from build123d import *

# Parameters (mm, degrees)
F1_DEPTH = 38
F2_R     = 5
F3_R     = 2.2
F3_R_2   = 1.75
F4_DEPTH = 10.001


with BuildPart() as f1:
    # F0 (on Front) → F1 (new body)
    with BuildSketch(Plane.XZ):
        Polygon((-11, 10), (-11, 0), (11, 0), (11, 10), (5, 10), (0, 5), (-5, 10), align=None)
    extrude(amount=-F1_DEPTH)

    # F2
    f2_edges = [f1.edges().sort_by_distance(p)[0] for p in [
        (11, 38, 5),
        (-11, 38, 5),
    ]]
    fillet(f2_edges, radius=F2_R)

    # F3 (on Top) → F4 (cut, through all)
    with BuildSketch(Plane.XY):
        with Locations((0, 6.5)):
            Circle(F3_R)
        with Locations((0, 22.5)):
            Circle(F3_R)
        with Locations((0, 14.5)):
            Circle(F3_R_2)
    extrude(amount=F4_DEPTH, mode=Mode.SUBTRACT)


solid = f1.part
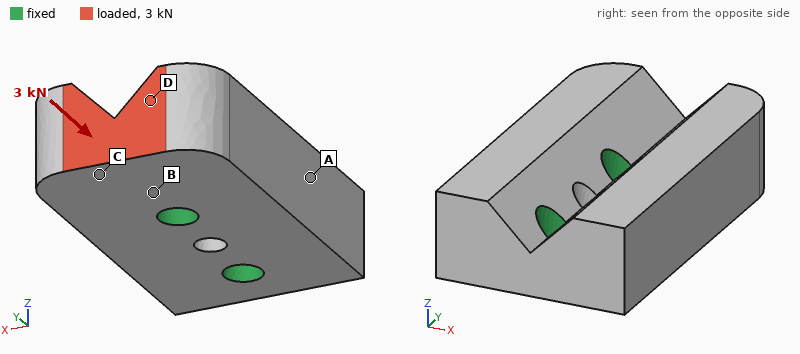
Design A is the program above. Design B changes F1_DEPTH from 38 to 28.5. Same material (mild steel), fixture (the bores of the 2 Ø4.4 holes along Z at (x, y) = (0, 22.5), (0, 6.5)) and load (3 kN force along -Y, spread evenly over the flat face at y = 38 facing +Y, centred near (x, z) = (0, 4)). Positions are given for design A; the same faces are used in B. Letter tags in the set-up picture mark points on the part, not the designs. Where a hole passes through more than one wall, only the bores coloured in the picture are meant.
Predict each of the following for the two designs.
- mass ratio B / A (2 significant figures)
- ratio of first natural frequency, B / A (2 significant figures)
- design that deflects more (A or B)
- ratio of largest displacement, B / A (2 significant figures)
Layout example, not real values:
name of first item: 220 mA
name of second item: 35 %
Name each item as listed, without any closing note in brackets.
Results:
mass ratio B / A: 0.74
ratio of first natural frequency, B / A: 1.5
design that deflects more: A
ratio of largest displacement, B / A: 0.58
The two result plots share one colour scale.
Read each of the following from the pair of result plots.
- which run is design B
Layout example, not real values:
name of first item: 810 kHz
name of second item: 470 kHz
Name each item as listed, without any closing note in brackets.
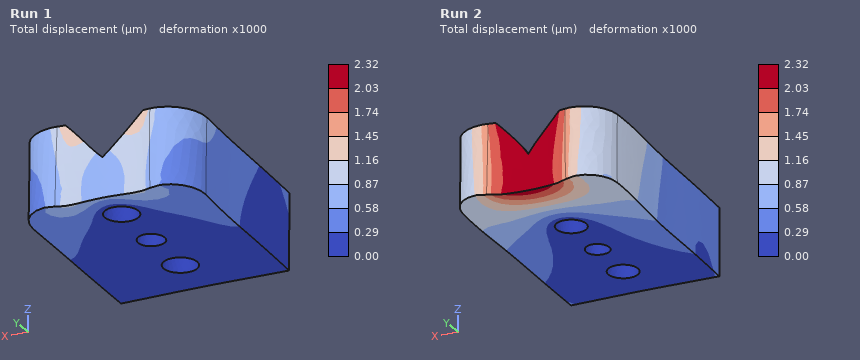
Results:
which run is design B: Run 1
